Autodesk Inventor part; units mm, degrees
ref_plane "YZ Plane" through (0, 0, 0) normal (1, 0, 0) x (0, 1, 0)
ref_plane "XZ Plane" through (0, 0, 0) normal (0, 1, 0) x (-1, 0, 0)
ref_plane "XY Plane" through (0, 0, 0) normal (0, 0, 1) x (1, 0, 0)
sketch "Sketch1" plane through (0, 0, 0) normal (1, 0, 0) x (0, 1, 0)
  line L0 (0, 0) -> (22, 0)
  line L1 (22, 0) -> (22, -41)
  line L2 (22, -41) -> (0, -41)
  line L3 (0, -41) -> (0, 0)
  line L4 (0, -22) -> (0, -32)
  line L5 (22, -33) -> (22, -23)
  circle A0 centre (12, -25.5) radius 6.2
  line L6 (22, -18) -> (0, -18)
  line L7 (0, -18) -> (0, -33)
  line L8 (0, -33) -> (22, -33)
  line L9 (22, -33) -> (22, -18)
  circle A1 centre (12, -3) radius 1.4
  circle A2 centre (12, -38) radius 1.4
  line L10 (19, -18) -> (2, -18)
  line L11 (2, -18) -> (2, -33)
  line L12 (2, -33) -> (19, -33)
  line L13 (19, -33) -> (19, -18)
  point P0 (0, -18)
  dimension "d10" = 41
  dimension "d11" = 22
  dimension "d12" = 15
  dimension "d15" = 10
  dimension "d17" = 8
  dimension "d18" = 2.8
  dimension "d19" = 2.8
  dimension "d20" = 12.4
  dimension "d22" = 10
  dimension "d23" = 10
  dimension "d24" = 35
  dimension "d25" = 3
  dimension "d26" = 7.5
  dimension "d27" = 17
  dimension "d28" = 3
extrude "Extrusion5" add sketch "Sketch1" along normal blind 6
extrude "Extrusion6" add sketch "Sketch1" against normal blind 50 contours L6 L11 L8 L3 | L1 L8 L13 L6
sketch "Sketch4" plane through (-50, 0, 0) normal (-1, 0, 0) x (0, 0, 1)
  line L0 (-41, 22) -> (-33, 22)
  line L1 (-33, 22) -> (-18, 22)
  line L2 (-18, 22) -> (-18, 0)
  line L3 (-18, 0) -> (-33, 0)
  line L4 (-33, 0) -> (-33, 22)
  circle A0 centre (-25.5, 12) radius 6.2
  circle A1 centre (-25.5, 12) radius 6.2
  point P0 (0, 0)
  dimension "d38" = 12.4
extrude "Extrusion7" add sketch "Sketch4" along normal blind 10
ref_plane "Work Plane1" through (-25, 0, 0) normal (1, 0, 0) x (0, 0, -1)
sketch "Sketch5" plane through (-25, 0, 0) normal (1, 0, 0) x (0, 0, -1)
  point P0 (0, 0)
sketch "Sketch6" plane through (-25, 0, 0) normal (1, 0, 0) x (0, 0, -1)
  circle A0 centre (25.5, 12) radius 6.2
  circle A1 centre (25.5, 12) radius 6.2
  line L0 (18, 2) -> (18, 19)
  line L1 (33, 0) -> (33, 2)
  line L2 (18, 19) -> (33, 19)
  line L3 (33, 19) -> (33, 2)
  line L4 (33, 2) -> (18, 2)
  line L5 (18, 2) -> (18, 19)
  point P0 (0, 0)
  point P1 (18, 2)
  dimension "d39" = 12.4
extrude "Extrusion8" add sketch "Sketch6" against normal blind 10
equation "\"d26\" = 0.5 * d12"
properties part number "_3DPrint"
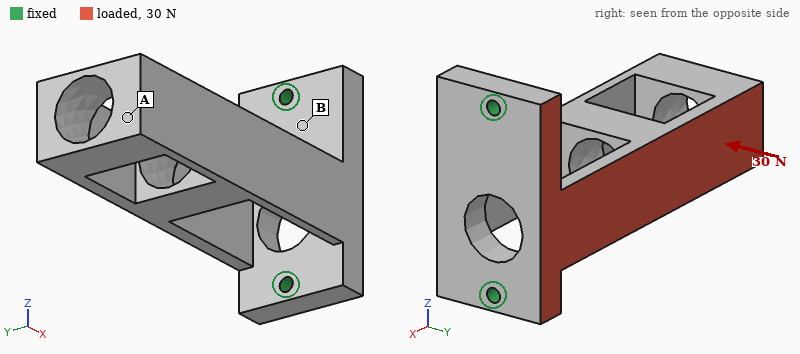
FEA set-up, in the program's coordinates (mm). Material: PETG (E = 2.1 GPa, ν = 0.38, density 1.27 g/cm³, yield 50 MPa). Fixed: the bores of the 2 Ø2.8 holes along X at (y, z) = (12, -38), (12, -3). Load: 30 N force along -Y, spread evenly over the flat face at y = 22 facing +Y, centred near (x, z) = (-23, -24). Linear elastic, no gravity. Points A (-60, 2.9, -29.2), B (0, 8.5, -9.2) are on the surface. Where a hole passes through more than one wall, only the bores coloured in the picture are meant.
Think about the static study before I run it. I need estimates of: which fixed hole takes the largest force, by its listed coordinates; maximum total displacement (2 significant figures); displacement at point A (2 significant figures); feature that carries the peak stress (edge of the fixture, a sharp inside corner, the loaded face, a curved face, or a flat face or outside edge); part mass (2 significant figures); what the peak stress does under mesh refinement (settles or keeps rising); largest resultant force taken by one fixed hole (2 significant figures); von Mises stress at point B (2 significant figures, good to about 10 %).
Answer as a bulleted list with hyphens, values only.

- (12, -38)
- 0.83 mm
- 0.83 mm
- edge of the fixture
- 15 g
- keeps rising
- 18 N
- 2.0 MPa
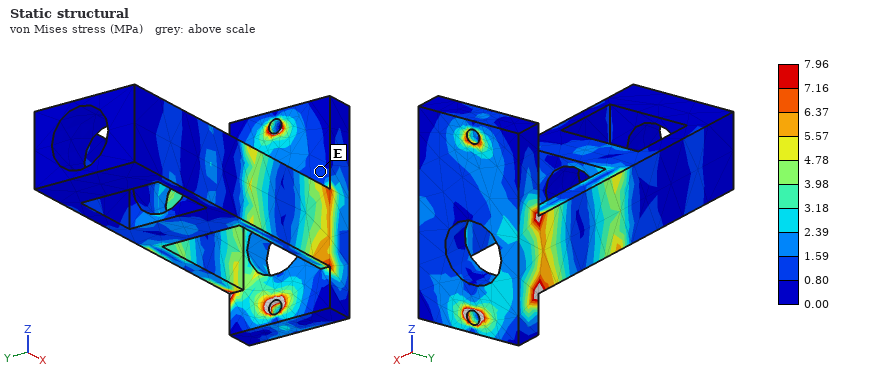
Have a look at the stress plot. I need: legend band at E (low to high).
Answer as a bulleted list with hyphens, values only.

- 0.80 to 1.59 MPa
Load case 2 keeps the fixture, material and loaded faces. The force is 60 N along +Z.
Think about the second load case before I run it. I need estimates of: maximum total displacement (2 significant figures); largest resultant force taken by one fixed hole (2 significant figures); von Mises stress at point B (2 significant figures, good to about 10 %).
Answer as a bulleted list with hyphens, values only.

- 0.96 mm
- 66 N
- 1.3 MPa
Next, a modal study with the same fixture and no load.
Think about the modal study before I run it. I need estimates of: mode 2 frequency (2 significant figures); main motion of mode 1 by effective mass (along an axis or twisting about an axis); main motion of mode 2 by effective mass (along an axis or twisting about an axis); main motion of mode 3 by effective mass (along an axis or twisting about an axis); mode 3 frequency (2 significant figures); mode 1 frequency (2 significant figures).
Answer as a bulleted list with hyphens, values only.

- 440 Hz
- along Y
- along Z
- twisting about X
- 1000 Hz
- 290 Hz
